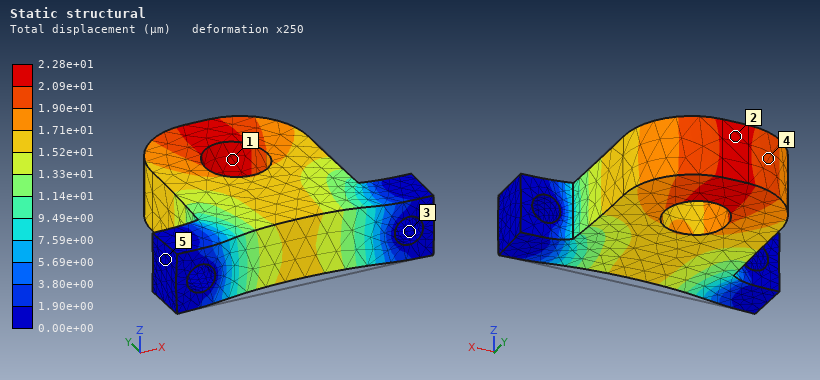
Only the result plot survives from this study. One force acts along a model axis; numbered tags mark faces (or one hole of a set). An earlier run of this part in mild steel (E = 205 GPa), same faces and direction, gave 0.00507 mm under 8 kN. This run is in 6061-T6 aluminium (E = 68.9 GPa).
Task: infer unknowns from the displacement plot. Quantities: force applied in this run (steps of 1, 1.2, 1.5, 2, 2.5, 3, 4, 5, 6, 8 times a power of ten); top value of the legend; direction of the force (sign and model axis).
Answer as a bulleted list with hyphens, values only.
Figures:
- 12 kN
- 2.28e+01 µm
- +Y
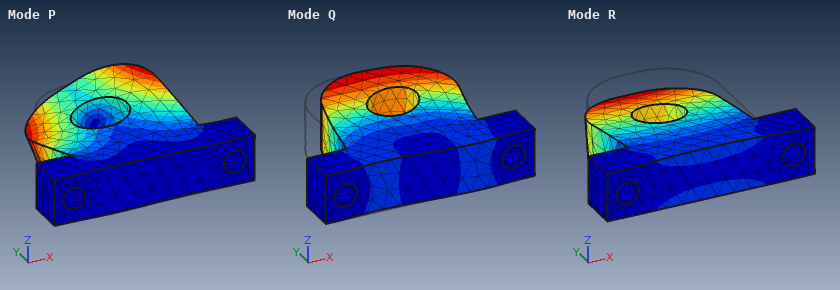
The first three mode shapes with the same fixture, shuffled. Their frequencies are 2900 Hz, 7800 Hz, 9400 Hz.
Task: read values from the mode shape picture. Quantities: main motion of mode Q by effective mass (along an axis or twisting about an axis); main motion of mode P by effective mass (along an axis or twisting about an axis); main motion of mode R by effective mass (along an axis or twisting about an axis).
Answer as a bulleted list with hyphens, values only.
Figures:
- along X
- twisting about Y
- along Z
